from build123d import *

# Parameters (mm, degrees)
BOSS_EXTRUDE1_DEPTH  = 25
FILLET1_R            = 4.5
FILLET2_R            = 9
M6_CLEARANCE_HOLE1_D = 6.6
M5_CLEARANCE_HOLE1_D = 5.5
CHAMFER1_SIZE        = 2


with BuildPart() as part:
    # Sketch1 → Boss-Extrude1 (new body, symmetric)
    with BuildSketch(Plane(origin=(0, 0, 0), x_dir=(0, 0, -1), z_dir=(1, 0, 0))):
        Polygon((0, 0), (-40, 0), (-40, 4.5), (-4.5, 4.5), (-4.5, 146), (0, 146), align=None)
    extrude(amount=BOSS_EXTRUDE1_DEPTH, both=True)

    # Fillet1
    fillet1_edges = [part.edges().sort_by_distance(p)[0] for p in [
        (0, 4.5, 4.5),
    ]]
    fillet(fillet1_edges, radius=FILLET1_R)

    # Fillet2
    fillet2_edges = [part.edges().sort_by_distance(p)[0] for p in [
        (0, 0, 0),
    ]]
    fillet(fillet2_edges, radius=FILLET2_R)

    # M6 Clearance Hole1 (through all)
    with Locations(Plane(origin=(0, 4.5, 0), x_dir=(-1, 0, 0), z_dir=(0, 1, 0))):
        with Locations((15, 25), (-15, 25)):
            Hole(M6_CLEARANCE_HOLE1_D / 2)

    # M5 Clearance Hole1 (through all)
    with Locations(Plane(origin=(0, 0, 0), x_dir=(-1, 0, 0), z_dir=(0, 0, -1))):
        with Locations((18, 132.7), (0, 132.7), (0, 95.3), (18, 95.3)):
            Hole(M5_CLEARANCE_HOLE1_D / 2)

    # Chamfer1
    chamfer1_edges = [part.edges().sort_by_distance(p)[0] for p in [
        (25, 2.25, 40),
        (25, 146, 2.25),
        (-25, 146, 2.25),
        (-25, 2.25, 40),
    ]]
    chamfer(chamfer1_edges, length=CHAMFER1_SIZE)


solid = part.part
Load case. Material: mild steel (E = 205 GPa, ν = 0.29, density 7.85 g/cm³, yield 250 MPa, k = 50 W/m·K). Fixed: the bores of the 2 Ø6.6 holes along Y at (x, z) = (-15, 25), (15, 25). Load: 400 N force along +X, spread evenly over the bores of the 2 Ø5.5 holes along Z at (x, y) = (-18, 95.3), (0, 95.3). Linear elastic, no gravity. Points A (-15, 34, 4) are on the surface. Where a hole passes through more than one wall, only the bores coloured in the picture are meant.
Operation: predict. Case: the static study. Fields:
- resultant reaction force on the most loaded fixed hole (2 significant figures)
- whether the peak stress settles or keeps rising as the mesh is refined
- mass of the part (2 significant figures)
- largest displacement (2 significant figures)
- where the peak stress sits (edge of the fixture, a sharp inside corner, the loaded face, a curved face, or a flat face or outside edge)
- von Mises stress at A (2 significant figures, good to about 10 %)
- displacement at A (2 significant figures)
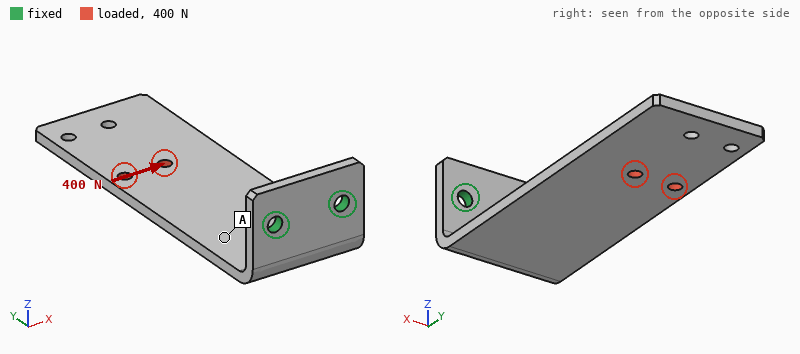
1.1 kN
keeps rising
310 g
0.38 mm
edge of the fixture
17 MPa
0.092 mm
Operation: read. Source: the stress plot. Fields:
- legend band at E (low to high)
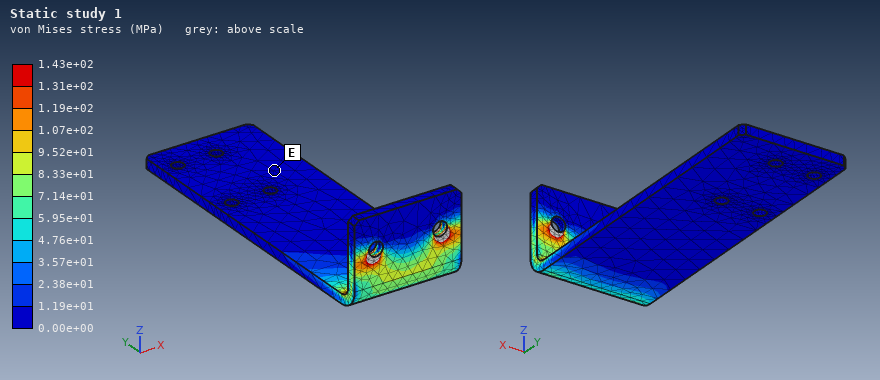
0.00e+00 to 1.19e+01 MPa
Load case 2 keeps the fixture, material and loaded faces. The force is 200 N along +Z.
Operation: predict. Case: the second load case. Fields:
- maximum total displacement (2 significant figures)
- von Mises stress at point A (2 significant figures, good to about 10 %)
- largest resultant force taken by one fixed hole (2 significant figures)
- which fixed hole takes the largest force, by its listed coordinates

1.9 mm
71 MPa
180 N
(-15, 25)
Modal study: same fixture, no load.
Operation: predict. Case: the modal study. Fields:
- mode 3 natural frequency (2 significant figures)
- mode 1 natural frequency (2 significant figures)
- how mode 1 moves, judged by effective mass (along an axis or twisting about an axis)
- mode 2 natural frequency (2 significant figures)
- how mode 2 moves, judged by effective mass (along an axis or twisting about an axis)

940 Hz
150 Hz
along Z
450 Hz
along X
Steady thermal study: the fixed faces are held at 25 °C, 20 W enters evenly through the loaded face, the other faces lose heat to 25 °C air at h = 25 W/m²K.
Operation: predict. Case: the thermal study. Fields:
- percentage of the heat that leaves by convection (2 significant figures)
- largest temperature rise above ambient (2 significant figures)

80 %
78 K
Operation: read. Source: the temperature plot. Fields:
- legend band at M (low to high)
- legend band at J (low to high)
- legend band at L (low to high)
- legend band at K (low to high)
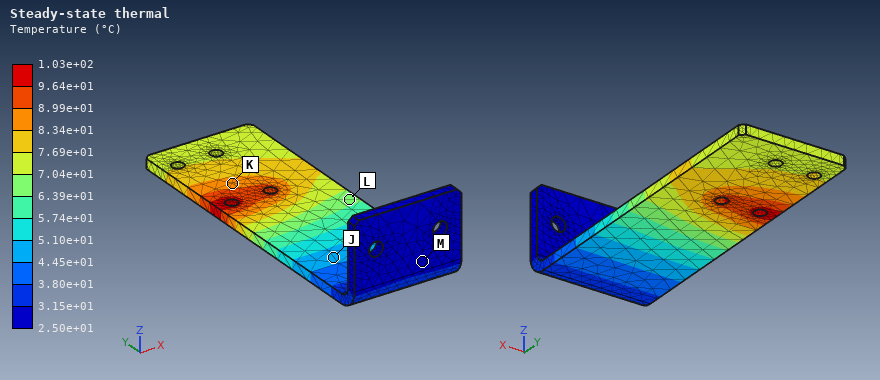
2.50e+01 to 3.15e+01 °C
4.45e+01 to 5.10e+01 °C
6.39e+01 to 7.04e+01 °C
8.34e+01 to 8.99e+01 °C
